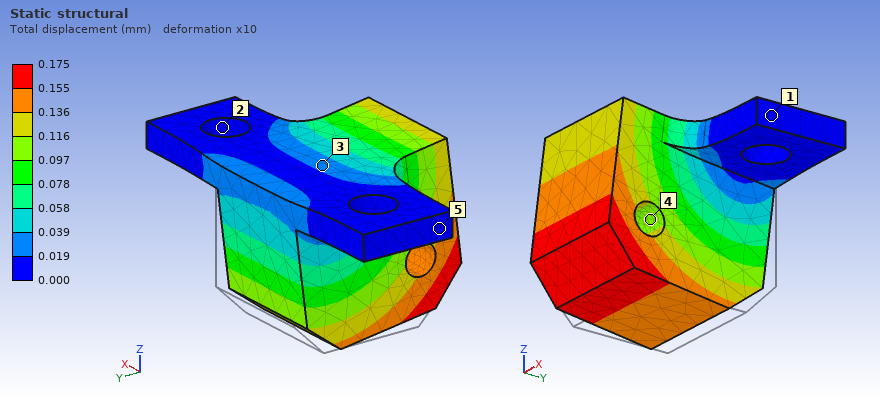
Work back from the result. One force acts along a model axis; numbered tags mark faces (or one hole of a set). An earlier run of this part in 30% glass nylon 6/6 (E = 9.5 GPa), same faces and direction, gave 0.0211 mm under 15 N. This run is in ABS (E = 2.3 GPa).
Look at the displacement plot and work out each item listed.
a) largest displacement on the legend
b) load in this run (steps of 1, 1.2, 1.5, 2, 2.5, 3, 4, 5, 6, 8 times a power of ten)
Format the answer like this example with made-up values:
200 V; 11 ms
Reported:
0.175 mm; 30 N
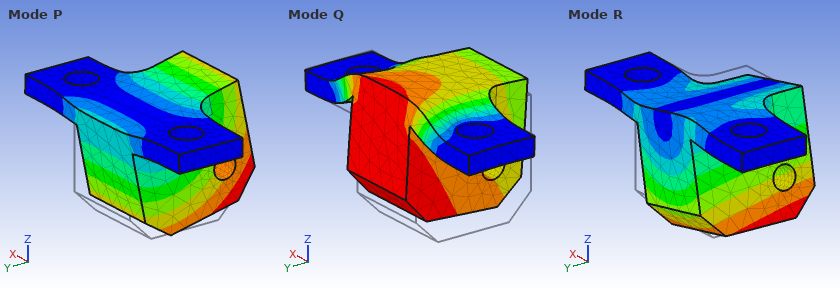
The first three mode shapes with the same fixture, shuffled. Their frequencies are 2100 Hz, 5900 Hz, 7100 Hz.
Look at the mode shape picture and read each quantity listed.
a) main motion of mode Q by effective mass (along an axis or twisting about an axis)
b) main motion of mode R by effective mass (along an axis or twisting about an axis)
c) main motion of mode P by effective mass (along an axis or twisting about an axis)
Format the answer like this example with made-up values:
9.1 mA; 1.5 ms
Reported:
along Z; along X; along Y
